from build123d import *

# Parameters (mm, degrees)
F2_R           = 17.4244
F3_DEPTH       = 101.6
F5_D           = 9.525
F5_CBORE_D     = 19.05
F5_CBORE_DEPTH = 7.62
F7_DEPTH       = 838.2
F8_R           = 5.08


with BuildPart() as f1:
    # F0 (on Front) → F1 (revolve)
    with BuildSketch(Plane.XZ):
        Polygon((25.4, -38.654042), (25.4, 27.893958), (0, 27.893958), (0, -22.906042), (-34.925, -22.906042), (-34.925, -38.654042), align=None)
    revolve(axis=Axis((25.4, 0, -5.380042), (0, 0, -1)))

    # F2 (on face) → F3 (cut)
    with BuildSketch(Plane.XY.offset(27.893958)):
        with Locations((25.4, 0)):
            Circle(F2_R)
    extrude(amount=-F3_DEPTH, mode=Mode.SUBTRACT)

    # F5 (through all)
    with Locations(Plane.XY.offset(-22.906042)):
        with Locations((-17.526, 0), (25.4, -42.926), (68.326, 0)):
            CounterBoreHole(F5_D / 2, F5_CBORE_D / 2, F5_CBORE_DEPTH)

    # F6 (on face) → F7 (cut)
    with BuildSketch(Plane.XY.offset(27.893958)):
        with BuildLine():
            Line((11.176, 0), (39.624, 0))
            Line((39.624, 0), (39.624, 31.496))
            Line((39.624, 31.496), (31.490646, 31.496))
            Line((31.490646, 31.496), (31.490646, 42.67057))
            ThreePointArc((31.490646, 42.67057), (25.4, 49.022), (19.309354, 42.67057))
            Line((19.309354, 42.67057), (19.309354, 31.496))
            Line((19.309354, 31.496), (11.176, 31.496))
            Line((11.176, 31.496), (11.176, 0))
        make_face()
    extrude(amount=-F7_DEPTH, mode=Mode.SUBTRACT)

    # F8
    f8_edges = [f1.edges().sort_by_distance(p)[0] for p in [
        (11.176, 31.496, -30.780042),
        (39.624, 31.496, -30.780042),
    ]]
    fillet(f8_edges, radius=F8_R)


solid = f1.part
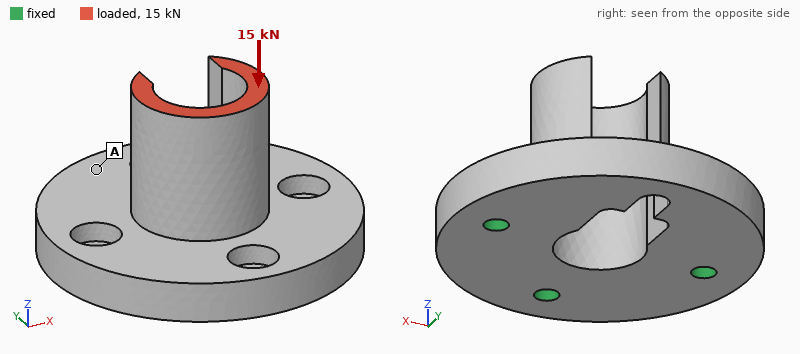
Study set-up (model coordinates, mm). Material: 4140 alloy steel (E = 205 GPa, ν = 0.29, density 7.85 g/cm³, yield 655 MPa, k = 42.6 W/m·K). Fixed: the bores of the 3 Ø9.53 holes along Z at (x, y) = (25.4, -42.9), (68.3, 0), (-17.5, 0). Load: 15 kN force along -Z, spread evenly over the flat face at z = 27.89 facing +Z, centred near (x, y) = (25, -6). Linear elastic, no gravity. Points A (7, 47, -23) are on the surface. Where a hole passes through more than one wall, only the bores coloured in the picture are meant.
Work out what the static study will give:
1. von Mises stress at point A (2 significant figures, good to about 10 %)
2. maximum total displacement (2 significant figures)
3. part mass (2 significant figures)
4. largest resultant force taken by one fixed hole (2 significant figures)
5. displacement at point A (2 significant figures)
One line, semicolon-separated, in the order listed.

17 MPa; 31 µm; 1.5 kg; 6.5 kN; 23 µm
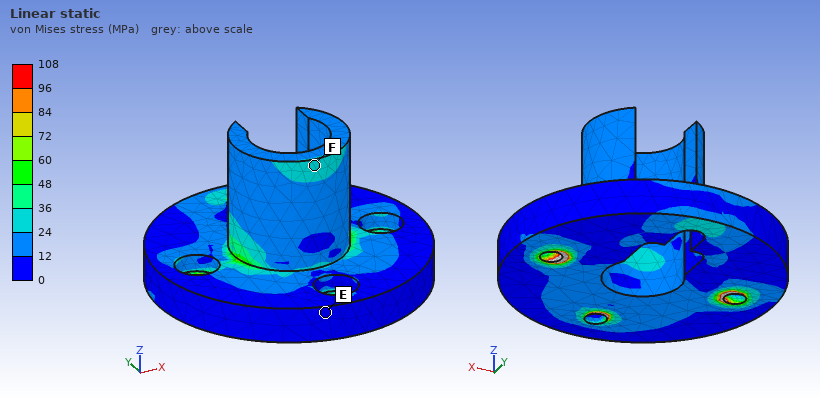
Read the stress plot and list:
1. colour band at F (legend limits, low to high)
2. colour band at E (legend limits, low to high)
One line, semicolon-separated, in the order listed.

24 to 36 MPa; 0 to 12 MPa
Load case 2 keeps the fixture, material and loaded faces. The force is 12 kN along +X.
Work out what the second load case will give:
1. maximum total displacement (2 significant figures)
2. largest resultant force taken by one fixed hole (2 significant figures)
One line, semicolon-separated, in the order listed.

0.23 mm; 11 kN
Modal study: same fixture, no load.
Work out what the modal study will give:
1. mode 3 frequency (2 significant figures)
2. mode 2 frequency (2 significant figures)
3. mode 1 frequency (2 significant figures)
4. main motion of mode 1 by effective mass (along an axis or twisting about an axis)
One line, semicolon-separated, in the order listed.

5200 Hz; 3900 Hz; 2600 Hz; along Z
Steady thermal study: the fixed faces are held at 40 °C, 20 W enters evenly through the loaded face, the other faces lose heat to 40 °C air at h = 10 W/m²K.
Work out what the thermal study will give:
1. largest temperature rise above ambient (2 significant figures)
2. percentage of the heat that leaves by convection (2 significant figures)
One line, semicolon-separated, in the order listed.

35 K; 17 %
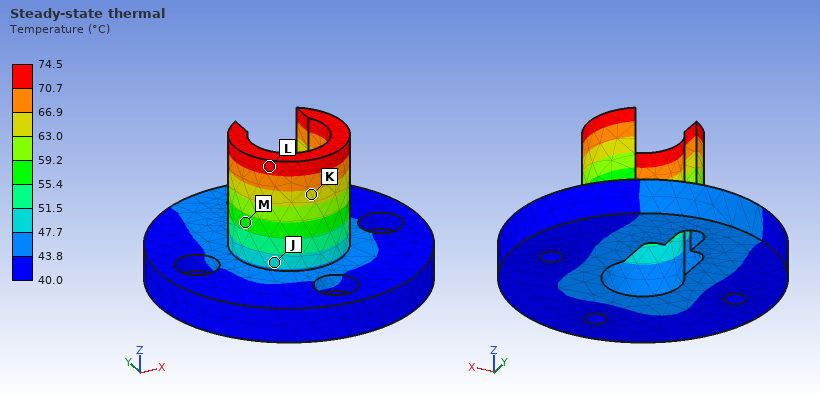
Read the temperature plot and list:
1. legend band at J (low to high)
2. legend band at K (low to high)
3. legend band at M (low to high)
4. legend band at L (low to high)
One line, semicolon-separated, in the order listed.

47.7 to 51.5 °C; 63.0 to 66.9 °C; 55.4 to 59.2 °C; 70.7 to 74.5 °C
